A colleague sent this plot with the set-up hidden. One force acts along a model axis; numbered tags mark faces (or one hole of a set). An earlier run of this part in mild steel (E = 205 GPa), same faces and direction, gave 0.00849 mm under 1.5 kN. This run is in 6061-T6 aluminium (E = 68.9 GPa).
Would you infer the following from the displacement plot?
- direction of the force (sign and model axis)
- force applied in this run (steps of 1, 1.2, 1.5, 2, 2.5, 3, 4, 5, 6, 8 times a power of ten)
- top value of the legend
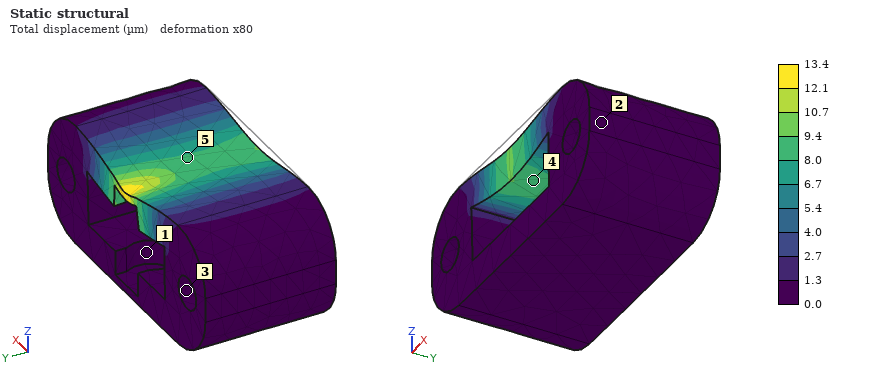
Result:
-Z
800 N
13.4 µm
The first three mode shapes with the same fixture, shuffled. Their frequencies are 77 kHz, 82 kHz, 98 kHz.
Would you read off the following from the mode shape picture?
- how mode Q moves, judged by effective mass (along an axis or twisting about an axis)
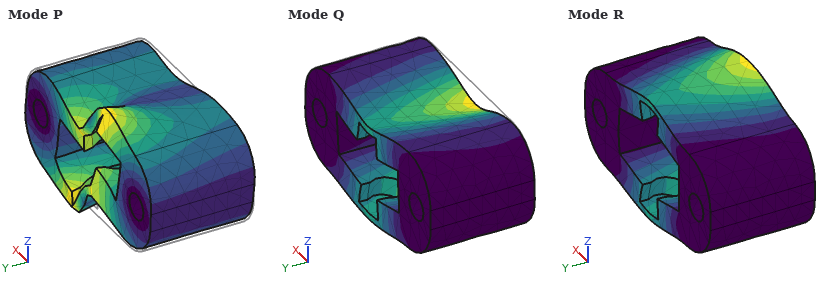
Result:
along Z
